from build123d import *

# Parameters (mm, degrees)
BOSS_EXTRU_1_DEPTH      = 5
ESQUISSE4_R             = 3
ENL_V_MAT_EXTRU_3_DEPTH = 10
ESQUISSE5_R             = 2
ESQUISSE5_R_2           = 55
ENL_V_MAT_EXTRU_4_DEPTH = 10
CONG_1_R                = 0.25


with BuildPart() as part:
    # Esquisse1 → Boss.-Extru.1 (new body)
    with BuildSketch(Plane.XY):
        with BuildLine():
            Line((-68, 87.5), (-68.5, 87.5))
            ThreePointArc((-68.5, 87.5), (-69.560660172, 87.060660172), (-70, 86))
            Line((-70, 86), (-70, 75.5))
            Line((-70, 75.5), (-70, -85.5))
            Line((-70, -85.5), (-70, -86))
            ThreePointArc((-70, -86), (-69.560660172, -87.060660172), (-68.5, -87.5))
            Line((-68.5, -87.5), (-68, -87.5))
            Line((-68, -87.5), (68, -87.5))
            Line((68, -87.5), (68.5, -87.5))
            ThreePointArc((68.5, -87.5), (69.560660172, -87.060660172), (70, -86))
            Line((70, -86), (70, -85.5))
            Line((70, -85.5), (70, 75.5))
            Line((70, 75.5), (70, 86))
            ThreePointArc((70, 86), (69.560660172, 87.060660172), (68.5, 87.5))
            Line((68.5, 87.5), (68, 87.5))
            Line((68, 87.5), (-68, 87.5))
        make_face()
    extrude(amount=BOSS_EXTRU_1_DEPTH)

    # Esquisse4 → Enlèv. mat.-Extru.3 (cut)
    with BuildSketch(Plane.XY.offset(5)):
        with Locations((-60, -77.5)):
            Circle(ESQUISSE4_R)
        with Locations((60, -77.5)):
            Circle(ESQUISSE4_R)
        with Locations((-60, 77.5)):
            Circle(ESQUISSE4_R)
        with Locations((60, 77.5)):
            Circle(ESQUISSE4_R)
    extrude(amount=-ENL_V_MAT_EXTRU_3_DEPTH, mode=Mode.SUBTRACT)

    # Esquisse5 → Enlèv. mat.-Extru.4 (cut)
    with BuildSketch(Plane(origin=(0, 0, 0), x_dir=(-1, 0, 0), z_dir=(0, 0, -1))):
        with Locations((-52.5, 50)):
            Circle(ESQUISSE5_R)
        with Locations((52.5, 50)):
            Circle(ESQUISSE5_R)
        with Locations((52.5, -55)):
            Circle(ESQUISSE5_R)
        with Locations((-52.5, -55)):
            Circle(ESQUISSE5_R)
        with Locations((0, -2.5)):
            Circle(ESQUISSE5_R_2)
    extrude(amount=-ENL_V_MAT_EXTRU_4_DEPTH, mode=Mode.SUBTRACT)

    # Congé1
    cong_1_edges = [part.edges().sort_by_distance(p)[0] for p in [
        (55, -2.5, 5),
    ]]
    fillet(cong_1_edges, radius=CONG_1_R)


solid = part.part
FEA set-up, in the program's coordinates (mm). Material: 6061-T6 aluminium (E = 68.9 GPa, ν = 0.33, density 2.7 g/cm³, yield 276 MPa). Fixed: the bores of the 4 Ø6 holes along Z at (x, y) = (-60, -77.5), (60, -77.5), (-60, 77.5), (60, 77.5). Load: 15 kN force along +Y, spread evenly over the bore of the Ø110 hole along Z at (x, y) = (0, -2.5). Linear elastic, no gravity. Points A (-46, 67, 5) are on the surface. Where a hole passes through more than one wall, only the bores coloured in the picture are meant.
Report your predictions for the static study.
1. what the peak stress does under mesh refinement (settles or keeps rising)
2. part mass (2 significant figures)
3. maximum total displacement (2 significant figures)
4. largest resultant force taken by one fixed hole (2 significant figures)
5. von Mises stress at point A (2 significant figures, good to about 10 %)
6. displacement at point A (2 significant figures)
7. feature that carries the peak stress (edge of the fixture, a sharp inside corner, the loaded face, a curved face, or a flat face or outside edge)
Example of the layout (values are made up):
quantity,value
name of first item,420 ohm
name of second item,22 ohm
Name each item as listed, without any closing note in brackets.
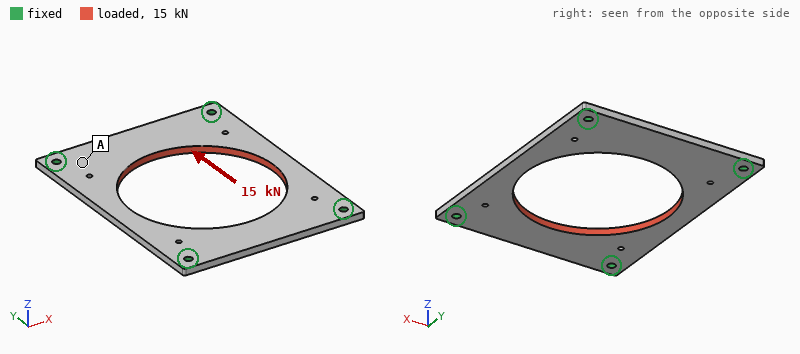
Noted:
quantity,value
what the peak stress does under mesh refinement,keeps rising
part mass,200 g
maximum total displacement,59 µm
largest resultant force taken by one fixed hole,4.0 kN
von Mises stress at point A,22 MPa
displacement at point A,16 µm
feature that carries the peak stress,edge of the fixture
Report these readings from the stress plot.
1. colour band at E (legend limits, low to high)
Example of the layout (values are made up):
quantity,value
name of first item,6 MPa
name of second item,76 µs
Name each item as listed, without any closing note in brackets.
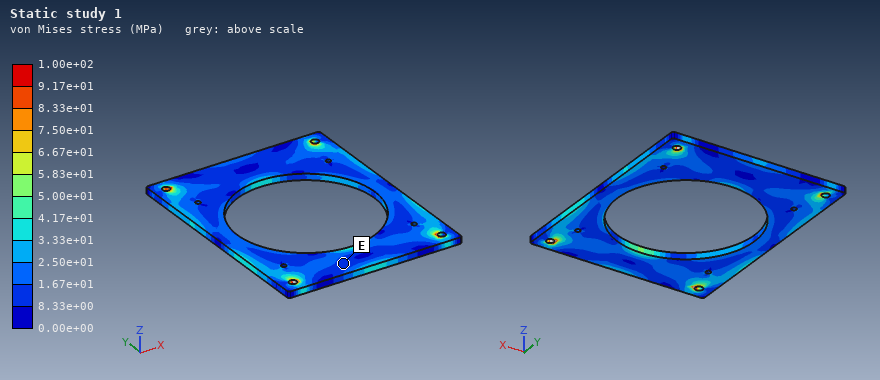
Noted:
quantity,value
colour band at E,8.33e+00 to 1.67e+01 MPa
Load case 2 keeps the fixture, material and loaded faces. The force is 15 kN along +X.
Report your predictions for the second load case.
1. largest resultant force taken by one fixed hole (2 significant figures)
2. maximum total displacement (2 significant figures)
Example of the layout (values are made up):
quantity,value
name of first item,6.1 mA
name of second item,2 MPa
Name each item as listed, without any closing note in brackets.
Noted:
quantity,value
largest resultant force taken by one fixed hole,4.0 kN
maximum total displacement,100 µm
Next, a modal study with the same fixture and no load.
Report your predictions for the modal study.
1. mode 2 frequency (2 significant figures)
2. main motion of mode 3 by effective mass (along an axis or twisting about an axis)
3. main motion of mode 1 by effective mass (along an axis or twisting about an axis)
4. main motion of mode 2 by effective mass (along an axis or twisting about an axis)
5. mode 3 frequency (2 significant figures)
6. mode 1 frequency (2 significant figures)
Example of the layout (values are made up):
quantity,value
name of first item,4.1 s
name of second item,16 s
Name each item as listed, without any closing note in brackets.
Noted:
quantity,value
mode 2 frequency,1300 Hz
main motion of mode 3 by effective mass,along Z
main motion of mode 1 by effective mass,along Z
main motion of mode 2 by effective mass,twisting about Y
mode 3 frequency,1700 Hz
mode 1 frequency,1200 Hz
